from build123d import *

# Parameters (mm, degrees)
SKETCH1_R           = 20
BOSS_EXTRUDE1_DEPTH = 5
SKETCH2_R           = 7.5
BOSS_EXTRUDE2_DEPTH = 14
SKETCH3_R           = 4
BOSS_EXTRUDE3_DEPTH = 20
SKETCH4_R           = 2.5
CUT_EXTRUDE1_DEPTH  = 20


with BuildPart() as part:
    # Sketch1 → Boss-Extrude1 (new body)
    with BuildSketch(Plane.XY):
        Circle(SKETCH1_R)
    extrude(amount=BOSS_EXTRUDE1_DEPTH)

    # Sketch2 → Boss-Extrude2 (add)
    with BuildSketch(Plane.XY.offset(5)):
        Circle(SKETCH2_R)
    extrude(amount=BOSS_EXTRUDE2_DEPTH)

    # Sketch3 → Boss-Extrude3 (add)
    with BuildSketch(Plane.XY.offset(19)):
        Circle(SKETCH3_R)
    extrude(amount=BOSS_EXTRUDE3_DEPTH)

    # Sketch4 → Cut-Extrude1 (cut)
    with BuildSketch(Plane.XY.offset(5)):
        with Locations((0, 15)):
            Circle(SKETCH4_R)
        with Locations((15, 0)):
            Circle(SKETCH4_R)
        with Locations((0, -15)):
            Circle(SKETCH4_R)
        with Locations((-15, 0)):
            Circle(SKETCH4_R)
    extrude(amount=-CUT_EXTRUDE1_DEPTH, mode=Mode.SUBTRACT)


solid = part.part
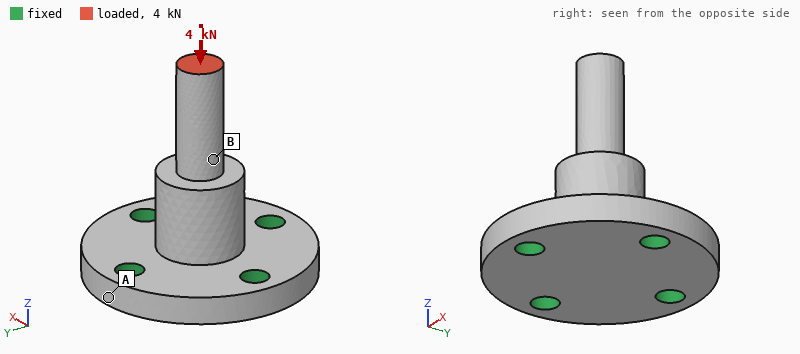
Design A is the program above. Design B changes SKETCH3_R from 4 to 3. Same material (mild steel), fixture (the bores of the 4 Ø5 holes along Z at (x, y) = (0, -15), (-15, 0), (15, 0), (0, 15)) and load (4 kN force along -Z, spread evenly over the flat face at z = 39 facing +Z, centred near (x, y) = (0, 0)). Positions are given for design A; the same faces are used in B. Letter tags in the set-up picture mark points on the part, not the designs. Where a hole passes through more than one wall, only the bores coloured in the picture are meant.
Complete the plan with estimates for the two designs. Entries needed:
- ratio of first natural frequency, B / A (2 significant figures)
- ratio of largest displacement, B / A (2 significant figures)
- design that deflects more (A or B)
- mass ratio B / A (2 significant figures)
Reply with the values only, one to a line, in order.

0.96
1.5
B
0.95
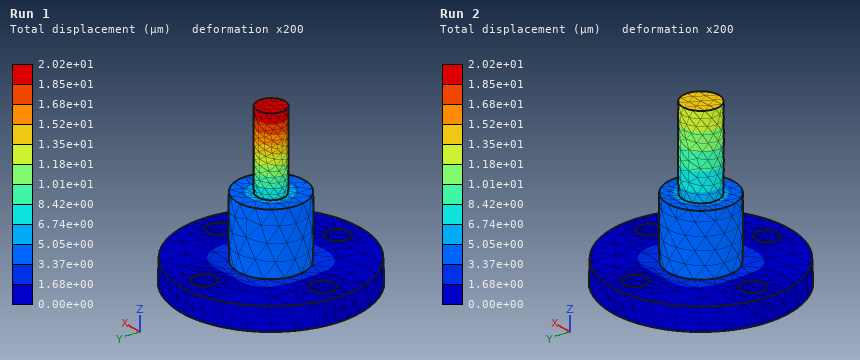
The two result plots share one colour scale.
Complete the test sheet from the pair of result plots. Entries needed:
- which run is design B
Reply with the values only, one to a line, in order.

Run 1
